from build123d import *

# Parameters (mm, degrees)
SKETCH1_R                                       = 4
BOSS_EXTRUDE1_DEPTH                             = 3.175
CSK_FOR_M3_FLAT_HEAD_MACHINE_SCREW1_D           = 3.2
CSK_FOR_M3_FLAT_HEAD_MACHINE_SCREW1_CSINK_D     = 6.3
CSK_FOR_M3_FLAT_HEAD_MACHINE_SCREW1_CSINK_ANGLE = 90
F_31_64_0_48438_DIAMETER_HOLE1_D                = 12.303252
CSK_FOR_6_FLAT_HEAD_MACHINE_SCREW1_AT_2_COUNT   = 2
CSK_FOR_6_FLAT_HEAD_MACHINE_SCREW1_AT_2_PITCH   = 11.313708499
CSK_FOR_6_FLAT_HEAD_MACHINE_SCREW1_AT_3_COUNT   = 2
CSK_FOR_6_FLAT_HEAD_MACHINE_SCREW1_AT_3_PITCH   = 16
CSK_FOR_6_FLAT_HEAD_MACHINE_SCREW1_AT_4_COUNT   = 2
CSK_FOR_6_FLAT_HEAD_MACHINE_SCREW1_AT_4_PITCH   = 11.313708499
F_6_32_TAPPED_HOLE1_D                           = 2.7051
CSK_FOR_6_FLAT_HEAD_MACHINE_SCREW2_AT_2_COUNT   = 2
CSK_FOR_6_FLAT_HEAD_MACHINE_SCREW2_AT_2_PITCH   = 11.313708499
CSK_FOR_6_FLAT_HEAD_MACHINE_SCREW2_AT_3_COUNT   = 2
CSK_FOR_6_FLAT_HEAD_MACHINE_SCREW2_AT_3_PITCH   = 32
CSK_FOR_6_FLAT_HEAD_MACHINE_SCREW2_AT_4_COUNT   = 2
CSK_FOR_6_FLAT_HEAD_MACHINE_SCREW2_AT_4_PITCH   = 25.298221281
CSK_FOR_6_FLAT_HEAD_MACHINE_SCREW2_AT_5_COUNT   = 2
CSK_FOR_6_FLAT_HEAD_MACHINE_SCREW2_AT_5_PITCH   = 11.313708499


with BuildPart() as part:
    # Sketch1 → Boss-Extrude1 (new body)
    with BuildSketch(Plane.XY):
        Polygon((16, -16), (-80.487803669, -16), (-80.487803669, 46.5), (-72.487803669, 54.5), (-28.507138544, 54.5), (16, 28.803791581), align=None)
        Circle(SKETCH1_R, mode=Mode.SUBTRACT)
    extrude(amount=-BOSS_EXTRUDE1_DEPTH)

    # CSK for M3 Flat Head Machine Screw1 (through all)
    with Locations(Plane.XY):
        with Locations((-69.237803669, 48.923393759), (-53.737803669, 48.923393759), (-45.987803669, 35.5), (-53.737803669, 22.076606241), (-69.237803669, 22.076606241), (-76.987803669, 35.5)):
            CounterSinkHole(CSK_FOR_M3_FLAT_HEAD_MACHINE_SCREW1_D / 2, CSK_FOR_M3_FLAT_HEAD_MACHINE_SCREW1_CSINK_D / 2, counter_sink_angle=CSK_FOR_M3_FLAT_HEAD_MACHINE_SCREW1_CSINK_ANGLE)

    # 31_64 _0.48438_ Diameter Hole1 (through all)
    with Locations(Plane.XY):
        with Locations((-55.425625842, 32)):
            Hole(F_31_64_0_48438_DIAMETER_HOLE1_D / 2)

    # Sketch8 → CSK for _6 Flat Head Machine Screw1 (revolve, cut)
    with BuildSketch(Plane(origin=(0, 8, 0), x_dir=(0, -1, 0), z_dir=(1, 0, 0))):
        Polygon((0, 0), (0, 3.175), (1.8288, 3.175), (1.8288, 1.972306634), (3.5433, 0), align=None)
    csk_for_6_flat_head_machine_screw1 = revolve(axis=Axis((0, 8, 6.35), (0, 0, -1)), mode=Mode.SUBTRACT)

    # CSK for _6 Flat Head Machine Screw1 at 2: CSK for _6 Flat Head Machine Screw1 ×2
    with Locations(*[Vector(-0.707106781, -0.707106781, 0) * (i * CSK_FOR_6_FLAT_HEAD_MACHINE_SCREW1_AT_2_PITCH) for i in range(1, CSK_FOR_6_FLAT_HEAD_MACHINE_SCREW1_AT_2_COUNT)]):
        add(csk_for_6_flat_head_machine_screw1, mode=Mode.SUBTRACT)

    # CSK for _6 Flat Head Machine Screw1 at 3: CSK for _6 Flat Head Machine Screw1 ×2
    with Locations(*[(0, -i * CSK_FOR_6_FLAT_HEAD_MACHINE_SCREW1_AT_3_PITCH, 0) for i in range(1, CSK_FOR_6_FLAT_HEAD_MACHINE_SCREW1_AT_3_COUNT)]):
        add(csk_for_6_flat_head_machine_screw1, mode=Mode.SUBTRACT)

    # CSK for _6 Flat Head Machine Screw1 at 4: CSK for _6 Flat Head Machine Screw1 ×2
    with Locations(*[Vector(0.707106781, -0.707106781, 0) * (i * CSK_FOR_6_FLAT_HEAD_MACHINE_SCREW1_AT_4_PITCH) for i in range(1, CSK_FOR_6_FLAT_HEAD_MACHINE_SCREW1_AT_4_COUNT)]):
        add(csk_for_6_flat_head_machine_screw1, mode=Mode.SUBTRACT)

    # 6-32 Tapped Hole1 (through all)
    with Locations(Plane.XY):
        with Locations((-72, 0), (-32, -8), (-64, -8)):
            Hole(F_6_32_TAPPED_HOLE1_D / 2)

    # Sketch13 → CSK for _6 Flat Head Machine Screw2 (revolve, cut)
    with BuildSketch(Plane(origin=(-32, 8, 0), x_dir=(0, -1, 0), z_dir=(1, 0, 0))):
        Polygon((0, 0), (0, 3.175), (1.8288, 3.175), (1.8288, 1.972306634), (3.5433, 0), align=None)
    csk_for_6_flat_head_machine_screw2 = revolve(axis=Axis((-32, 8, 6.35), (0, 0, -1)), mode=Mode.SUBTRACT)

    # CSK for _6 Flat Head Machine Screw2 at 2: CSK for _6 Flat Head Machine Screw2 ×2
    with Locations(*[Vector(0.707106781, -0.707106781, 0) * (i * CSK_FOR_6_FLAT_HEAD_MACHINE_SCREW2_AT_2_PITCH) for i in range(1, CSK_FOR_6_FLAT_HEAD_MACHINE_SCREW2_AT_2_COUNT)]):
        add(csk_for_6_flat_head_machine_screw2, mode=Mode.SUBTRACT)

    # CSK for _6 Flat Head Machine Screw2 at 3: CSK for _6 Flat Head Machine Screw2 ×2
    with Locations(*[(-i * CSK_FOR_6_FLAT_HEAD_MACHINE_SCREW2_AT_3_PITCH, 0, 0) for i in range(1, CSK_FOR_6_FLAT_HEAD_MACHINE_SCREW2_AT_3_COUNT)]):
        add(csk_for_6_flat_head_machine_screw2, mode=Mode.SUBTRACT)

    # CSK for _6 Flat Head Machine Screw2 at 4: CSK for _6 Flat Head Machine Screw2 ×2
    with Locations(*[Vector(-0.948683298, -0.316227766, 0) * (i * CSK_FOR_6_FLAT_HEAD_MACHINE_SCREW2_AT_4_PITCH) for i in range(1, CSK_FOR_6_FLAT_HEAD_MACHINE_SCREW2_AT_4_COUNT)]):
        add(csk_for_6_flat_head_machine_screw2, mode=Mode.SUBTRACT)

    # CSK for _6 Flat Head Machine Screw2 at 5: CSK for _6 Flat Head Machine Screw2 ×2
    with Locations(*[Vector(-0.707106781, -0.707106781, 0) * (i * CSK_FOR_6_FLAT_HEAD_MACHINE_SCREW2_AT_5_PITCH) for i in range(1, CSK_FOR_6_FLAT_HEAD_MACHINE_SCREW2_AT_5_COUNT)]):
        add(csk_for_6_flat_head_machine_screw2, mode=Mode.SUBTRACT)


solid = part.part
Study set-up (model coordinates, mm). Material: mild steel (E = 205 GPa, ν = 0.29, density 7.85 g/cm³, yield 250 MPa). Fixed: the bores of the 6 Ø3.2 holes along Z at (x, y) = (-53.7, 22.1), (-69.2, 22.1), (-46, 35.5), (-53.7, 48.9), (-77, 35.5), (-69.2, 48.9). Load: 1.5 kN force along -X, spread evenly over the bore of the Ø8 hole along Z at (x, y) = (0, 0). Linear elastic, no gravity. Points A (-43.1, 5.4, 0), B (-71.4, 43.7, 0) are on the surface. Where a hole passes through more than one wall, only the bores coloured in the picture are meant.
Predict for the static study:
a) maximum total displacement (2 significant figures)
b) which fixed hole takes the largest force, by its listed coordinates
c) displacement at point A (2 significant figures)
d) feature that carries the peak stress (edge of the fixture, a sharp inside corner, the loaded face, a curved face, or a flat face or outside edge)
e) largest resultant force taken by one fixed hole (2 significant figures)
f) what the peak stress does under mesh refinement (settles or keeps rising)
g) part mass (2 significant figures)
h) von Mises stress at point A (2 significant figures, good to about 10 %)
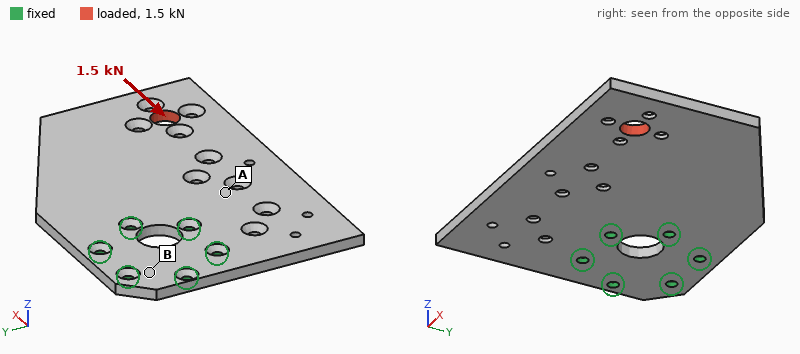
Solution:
21 µm
(-53.7, 22.1)
5.5 µm
edge of the fixture
1.2 kN
keeps rising
140 g
18 MPa
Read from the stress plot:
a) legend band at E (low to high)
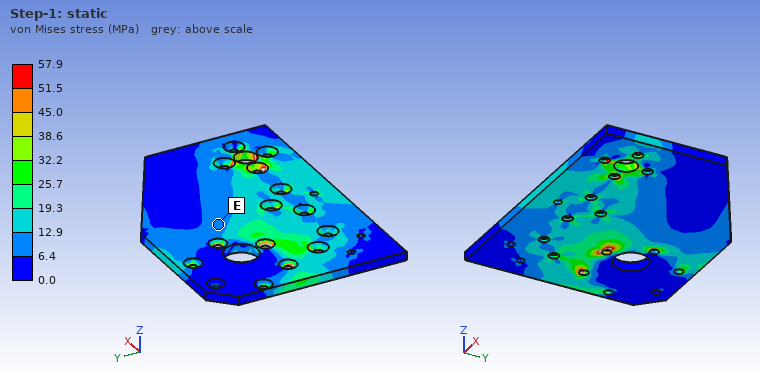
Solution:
6.4 to 12.9 MPa
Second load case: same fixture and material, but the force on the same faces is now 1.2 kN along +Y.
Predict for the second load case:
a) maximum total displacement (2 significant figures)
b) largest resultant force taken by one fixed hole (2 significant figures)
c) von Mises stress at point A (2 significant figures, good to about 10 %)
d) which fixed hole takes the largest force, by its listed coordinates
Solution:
24 µm
1.3 kN
12 MPa
(-46, 35.5)
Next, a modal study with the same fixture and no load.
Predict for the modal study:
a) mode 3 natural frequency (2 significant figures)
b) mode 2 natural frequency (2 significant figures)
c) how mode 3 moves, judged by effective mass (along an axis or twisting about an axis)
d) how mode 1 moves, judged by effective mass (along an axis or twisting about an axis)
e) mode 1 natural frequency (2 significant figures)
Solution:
2100 Hz
1300 Hz
along Z
along Z
560 Hz
